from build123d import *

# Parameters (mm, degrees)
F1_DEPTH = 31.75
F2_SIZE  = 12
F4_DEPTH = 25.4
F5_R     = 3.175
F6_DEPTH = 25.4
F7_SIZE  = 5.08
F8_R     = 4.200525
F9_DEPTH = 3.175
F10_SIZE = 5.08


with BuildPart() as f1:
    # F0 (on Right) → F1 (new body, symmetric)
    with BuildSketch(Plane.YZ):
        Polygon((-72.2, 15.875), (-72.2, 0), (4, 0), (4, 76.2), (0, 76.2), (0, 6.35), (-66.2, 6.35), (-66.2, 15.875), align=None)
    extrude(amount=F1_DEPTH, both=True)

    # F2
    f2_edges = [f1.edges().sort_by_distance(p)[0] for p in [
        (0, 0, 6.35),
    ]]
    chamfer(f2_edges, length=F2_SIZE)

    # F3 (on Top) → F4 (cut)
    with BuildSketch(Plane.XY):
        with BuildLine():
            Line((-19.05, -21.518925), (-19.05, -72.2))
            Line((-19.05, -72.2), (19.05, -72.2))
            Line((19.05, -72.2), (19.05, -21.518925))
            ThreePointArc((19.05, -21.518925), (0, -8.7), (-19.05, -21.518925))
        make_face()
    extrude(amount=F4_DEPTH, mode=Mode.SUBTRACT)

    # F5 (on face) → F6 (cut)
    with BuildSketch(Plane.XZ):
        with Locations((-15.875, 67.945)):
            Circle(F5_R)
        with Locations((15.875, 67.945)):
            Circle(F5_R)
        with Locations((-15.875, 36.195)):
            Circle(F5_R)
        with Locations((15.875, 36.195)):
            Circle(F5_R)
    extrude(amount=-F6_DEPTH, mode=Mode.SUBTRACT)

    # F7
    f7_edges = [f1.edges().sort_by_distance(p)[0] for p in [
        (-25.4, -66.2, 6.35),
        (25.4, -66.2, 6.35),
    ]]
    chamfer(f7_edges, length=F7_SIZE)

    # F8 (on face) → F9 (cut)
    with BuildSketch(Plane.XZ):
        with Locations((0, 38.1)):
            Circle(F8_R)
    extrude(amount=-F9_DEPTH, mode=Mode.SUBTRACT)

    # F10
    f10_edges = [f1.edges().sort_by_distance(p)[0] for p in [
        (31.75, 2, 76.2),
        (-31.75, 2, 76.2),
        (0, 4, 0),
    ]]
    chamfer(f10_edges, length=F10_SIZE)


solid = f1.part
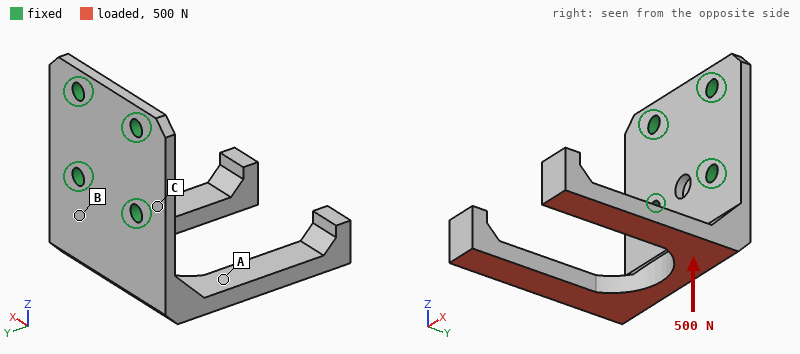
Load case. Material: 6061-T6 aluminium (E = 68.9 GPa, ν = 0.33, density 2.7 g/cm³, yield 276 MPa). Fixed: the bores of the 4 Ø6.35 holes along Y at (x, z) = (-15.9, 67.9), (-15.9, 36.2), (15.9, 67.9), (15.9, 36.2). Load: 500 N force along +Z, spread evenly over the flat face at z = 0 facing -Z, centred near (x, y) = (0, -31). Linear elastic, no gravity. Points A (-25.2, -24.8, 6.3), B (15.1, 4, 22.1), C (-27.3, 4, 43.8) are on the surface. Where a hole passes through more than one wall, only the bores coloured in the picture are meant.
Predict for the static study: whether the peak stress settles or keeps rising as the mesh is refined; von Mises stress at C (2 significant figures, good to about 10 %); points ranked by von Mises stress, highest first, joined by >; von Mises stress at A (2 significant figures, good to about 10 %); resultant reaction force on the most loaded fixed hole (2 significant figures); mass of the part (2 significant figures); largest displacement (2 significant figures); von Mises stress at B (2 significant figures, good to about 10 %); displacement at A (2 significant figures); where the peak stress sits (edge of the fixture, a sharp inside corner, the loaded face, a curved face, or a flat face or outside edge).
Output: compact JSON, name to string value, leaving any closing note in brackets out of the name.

{"whether the peak stress settles or keeps rising as the mesh is refined": "keeps rising", "von Mises stress at C": "13 MPa", "points ranked by von Mises stress, highest first, joined by >": "B > A > C", "von Mises stress at A": "37 MPa", "resultant reaction force on the most loaded fixed hole": "250 N", "mass of the part": "100 g", "largest displacement": "1.3 mm", "von Mises stress at B": "84 MPa", "displacement at A": "0.46 mm", "where the peak stress sits": "edge of the fixture"}
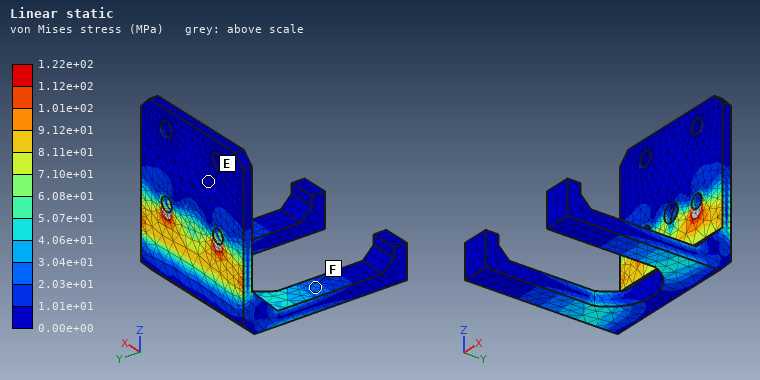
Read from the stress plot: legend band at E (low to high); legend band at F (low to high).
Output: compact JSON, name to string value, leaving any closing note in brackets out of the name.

{"legend band at E": "0.00e+00 to 1.01e+01 MPa", "legend band at F": "2.03e+01 to 3.04e+01 MPa"}
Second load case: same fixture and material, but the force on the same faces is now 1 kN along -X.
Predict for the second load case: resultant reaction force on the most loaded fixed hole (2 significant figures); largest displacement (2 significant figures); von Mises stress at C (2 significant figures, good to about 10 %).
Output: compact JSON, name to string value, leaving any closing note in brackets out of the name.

{"resultant reaction force on the most loaded fixed hole": "1.3 kN", "largest displacement": "0.53 mm", "von Mises stress at C": "33 MPa"}
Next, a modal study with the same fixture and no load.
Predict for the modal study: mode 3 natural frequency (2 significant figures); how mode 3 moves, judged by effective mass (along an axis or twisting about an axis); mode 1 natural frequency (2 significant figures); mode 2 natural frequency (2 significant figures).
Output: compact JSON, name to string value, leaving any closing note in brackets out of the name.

{"mode 3 natural frequency": "1100 Hz", "how mode 3 moves, judged by effective mass": "along X", "mode 1 natural frequency": "490 Hz", "mode 2 natural frequency": "910 Hz"}
